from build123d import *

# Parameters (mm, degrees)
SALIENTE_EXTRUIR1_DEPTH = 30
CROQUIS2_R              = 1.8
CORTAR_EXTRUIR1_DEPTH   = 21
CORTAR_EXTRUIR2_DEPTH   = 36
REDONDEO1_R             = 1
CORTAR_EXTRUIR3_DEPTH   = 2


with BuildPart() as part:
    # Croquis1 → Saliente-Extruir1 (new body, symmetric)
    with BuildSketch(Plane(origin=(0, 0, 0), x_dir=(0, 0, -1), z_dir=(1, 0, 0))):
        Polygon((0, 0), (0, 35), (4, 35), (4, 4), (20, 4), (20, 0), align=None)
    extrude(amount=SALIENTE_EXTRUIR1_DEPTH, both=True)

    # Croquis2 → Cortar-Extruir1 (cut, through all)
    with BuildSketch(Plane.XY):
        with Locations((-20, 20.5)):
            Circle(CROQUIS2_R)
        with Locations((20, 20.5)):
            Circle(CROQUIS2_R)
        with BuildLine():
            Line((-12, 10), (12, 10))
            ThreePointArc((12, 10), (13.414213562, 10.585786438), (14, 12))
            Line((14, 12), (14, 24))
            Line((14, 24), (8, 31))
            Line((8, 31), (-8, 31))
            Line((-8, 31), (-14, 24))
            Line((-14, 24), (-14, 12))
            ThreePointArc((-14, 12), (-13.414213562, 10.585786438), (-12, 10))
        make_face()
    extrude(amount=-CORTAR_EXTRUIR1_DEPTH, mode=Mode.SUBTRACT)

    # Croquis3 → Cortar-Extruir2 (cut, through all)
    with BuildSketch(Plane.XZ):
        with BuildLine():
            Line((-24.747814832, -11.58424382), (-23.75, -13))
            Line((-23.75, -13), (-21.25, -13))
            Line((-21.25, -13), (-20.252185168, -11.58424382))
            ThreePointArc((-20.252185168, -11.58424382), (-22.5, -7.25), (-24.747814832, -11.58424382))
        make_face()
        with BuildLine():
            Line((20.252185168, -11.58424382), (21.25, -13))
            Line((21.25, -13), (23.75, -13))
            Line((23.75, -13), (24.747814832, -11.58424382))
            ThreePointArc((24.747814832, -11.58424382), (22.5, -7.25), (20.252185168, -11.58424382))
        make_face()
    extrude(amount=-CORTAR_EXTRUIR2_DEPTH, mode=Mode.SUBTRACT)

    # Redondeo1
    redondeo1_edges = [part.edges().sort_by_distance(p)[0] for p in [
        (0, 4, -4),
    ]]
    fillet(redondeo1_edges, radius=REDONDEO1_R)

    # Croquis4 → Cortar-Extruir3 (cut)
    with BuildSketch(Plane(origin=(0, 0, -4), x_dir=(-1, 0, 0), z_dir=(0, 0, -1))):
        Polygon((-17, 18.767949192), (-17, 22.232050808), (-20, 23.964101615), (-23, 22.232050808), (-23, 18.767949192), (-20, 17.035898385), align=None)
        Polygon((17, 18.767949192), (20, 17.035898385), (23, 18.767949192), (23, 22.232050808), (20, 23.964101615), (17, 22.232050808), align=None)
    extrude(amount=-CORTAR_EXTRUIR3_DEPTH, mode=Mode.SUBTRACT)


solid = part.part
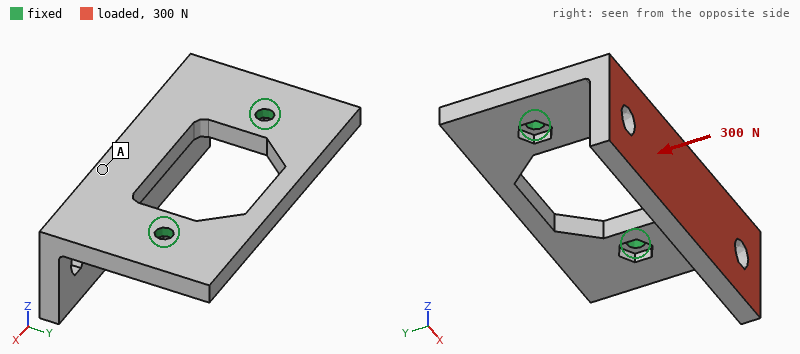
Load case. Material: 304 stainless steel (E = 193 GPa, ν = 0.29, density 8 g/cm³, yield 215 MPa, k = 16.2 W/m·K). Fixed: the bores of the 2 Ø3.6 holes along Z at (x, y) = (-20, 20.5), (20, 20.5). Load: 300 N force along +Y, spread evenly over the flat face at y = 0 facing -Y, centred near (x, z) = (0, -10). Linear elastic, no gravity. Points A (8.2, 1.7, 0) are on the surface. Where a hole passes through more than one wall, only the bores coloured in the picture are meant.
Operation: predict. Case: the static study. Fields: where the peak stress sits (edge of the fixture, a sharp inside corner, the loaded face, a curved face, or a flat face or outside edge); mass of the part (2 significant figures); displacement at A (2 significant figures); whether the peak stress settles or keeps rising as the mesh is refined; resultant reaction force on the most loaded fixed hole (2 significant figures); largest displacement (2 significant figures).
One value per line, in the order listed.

edge of the fixture
78 g
22 µm
keeps rising
160 N
44 µm
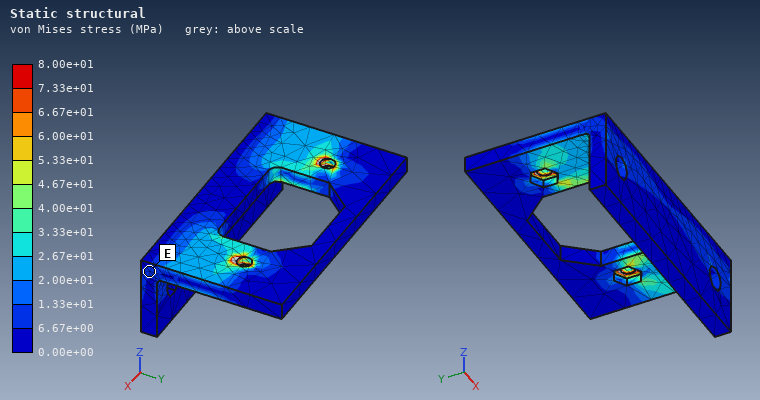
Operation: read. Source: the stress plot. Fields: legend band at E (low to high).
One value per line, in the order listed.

6.67e+00 to 1.33e+01 MPa
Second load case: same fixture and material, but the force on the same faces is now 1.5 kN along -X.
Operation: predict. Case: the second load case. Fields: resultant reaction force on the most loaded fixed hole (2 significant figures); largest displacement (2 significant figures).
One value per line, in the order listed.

1.0 kN
42 µm
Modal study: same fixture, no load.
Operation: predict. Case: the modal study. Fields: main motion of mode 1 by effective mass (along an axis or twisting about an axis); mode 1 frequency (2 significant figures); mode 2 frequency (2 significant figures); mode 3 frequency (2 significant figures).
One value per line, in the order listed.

along Z
1800 Hz
3700 Hz
6400 Hz
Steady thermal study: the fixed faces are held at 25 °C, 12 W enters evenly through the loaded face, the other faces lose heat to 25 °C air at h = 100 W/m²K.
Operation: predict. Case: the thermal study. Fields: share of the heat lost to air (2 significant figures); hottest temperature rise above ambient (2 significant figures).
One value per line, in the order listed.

81 %
45 K
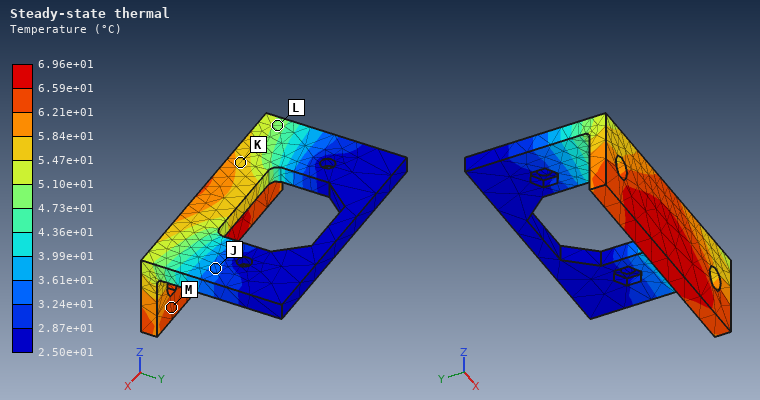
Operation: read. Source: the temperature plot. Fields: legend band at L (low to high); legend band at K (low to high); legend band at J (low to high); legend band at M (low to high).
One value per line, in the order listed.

4.73e+01 to 5.10e+01 °C
5.47e+01 to 5.84e+01 °C
3.24e+01 to 3.61e+01 °C
6.21e+01 to 6.59e+01 °C
